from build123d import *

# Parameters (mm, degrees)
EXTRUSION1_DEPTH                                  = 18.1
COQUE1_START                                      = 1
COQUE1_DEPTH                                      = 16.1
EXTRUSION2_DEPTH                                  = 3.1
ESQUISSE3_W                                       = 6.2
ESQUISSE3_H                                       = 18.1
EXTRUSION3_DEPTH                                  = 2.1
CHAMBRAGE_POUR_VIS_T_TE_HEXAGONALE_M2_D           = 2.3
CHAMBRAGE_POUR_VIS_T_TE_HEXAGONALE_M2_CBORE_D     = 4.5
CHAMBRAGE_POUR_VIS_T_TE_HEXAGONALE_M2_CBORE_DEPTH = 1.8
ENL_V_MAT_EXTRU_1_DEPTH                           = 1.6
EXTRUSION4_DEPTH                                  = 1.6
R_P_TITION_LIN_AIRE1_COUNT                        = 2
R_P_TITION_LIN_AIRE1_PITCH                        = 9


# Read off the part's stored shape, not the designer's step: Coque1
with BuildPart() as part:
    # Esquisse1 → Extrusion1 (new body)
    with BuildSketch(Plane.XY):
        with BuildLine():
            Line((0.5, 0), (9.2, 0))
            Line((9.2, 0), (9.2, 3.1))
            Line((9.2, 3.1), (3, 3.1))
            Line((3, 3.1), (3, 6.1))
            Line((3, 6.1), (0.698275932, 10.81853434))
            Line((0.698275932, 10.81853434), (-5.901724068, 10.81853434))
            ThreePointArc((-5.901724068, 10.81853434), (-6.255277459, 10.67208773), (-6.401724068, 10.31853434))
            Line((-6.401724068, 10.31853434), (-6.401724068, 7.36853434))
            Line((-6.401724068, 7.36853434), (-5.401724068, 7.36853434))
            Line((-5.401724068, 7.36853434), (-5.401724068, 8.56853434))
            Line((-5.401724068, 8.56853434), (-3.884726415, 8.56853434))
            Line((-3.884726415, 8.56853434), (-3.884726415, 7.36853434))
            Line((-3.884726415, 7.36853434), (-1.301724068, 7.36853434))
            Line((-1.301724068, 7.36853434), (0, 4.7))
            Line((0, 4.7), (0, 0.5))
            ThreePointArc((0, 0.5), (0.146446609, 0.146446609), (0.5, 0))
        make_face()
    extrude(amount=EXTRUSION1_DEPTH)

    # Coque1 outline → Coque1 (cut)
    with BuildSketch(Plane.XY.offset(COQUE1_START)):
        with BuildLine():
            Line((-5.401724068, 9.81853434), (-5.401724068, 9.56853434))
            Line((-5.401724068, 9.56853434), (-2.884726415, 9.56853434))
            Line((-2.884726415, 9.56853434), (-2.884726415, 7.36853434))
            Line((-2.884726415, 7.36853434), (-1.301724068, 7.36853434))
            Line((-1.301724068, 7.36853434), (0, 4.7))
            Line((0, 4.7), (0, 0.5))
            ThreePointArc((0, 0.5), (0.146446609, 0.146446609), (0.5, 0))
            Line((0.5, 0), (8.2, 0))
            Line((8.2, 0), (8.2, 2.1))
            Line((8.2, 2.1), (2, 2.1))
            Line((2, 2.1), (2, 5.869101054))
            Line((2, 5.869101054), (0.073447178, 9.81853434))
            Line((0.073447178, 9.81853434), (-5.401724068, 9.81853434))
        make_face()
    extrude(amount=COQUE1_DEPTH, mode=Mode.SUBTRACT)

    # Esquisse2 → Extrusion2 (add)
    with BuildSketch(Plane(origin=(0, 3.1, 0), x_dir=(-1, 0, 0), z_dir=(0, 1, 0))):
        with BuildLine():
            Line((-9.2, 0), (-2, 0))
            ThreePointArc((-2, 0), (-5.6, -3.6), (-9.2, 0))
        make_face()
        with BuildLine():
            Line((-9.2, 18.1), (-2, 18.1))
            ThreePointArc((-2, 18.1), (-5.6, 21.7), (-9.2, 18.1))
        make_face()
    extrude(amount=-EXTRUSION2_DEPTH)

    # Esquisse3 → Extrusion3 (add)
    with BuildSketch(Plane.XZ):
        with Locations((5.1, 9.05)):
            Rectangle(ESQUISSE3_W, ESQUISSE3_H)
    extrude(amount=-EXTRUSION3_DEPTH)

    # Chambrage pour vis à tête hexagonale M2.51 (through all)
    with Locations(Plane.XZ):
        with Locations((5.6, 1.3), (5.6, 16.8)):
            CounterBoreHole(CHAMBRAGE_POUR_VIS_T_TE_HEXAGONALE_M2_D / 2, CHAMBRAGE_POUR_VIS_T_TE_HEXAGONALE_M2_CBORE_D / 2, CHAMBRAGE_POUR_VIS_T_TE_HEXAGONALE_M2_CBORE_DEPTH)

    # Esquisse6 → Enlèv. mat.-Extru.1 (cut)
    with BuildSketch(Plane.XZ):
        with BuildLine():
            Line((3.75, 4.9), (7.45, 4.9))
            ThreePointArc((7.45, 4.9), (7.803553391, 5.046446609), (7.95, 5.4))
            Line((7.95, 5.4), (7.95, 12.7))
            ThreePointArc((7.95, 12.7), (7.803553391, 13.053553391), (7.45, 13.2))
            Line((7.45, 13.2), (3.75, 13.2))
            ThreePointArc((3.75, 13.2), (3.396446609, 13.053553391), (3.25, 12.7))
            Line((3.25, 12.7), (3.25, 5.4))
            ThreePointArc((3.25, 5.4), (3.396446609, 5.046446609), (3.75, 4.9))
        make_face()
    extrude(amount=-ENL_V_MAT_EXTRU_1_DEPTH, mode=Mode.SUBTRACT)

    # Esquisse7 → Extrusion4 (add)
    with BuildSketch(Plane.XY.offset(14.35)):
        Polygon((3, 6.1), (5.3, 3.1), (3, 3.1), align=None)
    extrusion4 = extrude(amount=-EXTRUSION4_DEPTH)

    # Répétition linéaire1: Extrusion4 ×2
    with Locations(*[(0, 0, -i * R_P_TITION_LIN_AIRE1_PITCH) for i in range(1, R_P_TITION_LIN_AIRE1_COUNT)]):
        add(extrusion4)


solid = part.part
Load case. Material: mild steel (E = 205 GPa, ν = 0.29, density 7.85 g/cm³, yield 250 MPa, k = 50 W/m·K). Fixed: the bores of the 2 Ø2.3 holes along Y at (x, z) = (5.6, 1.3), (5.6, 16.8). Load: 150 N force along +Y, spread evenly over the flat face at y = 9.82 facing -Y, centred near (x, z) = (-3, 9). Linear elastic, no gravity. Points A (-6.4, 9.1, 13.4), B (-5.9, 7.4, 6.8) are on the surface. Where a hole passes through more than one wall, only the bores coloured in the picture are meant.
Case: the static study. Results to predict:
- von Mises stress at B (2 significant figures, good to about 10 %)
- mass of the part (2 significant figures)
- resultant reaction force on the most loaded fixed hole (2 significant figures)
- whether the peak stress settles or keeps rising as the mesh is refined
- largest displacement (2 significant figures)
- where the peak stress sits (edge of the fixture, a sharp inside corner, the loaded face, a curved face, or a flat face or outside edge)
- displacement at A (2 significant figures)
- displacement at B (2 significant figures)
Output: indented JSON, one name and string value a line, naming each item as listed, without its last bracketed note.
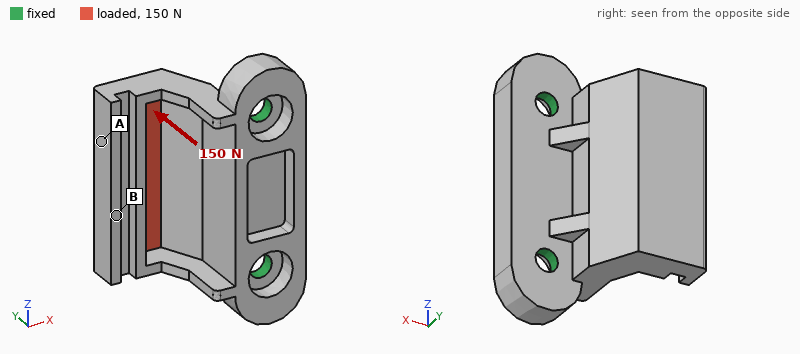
{
  "von Mises stress at B": "33 MPa",
  "mass of the part": "6.6 g",
  "resultant reaction force on the most loaded fixed hole": "76 N",
  "whether the peak stress settles or keeps rising as the mesh is refined": "keeps rising",
  "largest displacement": "42 µm",
  "where the peak stress sits": "edge of the fixture",
  "displacement at A": "39 µm",
  "displacement at B": "35 µm"
}
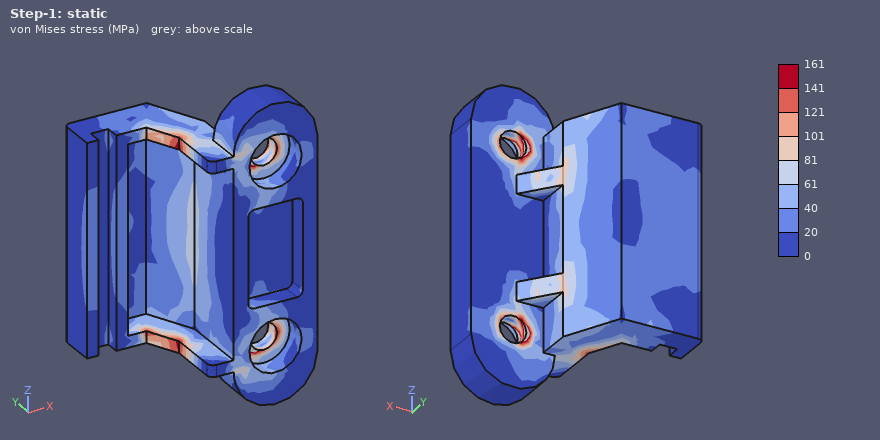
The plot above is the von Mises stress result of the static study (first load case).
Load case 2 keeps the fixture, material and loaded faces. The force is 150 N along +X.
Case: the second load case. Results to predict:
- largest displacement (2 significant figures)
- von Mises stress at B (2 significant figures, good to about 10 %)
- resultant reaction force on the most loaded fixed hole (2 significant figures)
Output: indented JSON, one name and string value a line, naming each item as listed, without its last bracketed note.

{
  "largest displacement": "37 µm",
  "von Mises stress at B": "12 MPa",
  "resultant reaction force on the most loaded fixed hole": "76 N"
}
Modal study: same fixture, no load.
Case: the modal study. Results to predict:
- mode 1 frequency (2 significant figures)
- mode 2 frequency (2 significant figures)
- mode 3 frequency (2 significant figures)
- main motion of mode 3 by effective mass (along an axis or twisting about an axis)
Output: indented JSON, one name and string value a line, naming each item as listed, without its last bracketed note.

{
  "mode 1 frequency": "6100 Hz",
  "mode 2 frequency": "9700 Hz",
  "mode 3 frequency": "21 kHz",
  "main motion of mode 3 by effective mass": "along X"
}
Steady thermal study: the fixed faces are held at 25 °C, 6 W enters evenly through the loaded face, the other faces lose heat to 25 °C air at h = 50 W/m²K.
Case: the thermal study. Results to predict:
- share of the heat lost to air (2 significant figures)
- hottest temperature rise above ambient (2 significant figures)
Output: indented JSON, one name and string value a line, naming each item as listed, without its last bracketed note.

{
  "share of the heat lost to air": "27 %",
  "hottest temperature rise above ambient": "54 K"
}
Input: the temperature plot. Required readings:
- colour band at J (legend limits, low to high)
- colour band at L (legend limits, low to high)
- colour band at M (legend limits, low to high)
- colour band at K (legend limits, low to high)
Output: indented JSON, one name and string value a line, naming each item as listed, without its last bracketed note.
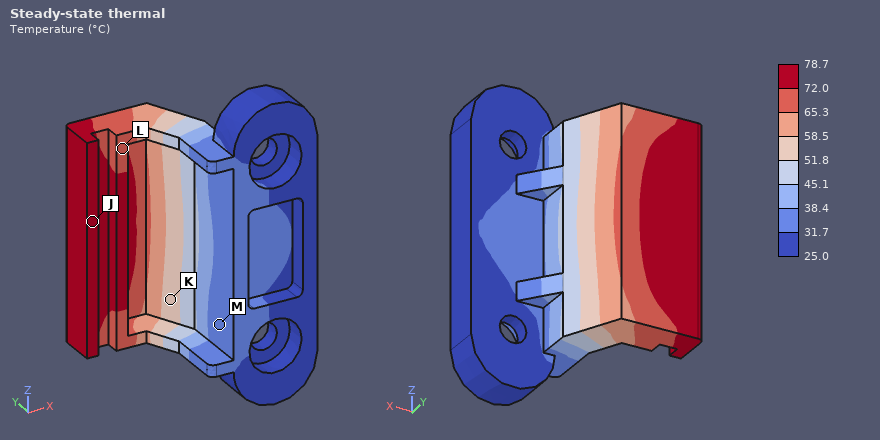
{
  "colour band at J": "72.0 to 78.7 °C",
  "colour band at L": "65.3 to 72.0 °C",
  "colour band at M": "31.7 to 38.4 °C",
  "colour band at K": "51.8 to 58.5 °C"
}
